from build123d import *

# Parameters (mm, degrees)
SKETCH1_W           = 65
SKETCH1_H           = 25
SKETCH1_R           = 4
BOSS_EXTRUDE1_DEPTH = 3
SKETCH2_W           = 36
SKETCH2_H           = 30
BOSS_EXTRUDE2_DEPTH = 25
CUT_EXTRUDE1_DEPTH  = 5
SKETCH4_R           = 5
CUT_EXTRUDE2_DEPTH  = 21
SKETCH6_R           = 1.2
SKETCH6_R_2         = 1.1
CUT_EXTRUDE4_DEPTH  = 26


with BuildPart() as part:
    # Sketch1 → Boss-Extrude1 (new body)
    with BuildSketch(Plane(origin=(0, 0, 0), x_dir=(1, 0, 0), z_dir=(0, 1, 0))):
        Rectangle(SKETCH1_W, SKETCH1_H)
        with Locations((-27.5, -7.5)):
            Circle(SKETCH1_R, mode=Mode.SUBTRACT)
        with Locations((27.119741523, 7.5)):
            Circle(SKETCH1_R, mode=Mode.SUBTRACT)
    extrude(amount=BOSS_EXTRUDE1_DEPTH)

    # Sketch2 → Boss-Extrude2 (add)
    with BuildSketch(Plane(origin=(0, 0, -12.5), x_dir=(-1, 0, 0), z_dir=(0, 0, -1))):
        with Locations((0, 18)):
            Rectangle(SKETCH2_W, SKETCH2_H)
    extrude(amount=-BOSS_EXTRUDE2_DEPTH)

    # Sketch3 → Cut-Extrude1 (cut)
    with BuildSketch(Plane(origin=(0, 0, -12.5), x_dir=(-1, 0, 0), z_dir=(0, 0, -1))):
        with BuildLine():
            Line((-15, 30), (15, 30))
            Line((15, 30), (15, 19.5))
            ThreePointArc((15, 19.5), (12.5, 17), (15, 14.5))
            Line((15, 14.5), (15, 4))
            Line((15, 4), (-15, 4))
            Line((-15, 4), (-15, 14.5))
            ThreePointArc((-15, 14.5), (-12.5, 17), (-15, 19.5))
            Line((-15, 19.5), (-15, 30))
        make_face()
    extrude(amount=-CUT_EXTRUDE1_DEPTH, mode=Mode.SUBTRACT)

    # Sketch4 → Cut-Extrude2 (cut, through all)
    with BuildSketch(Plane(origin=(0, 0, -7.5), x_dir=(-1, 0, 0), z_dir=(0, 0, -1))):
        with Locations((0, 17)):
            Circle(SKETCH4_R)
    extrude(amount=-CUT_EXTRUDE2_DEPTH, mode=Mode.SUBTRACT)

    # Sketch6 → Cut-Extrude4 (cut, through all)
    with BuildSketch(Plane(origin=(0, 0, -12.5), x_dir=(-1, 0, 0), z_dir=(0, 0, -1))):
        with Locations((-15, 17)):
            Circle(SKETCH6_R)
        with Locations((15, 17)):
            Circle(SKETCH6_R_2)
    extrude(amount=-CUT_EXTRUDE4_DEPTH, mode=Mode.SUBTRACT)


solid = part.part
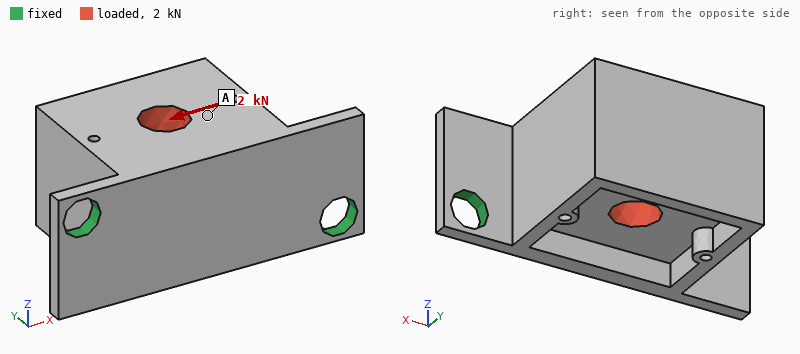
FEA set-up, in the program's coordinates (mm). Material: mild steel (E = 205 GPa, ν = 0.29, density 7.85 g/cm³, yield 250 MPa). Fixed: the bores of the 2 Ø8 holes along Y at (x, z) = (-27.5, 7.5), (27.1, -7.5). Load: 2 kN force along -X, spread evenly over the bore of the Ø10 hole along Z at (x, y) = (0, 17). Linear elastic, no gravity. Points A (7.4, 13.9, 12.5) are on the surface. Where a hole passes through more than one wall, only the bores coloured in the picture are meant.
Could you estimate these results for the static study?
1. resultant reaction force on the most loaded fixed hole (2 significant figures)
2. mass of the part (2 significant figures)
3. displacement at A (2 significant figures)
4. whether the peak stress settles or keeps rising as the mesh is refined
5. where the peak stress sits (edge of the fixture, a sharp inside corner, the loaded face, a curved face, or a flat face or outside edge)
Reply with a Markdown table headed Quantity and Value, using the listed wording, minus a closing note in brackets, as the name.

| Quantity | Value |
|---|---|
| resultant reaction force on the most loaded fixed hole | 1.2 kN |
| mass of the part | 200 g |
| displacement at A | 28 µm |
| whether the peak stress settles or keeps rising as the mesh is refined | keeps rising |
| where the peak stress sits | edge of the fixture |
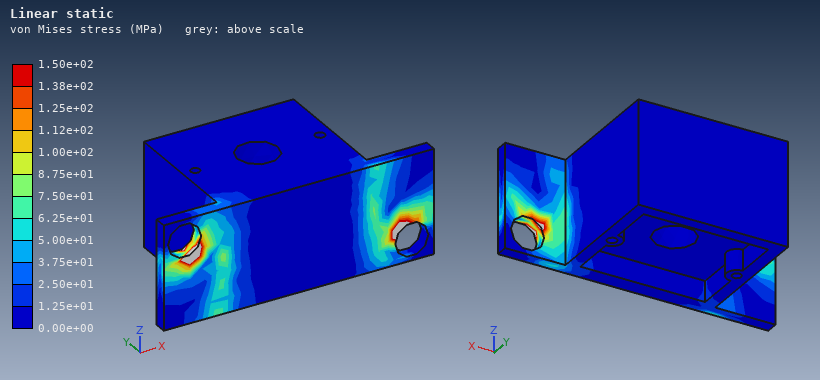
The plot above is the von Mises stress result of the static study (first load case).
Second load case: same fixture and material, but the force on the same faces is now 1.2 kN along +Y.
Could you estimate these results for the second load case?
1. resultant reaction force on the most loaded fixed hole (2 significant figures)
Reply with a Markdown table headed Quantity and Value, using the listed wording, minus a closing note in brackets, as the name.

| Quantity | Value |
|---|---|
| resultant reaction force on the most loaded fixed hole | 710 N |
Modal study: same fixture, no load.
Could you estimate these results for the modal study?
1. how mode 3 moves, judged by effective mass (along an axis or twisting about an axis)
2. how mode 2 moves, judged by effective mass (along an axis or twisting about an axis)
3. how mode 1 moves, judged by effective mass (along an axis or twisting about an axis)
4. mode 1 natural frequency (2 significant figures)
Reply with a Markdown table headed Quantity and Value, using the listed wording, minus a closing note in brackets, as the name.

| Quantity | Value |
|---|---|
| how mode 3 moves, judged by effective mass | along X |
| how mode 2 moves, judged by effective mass | along Y |
| how mode 1 moves, judged by effective mass | along Z |
| mode 1 natural frequency | 1400 Hz |
